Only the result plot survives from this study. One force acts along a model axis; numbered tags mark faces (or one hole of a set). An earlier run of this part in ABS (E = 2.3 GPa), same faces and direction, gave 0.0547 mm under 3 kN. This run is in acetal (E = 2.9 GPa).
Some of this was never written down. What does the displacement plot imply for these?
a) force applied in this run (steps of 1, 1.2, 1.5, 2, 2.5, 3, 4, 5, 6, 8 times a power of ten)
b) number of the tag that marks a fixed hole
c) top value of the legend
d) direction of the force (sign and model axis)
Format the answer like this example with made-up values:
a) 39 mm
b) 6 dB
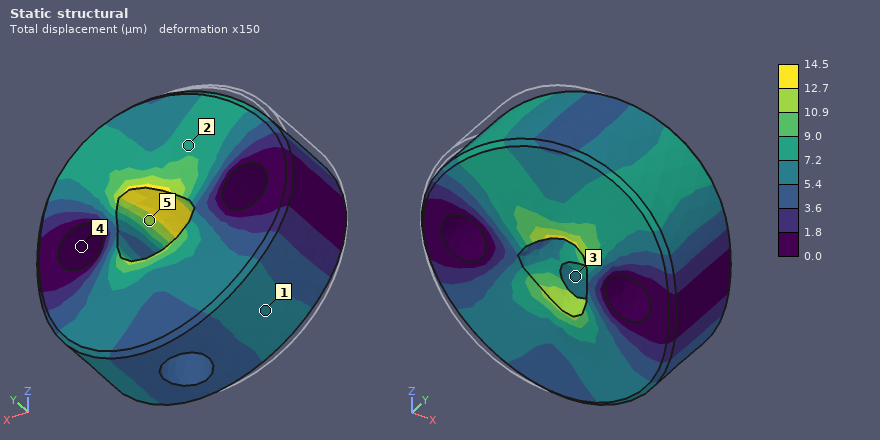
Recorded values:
a) 1 kN
b) 4
c) 14.5 µm
d) +X
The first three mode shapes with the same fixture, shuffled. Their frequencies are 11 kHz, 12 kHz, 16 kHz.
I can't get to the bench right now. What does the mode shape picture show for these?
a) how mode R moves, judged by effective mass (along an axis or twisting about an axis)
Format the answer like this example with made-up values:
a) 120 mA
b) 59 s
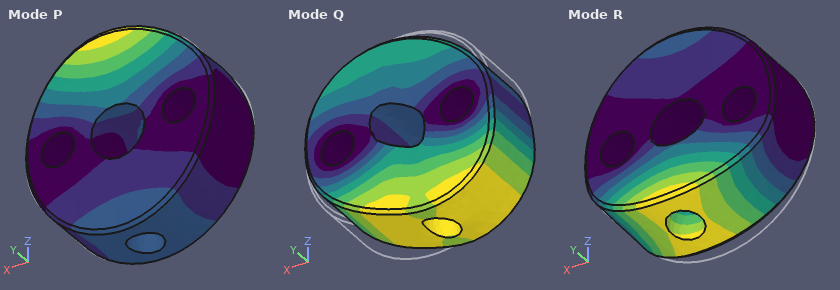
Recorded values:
a) along Y
